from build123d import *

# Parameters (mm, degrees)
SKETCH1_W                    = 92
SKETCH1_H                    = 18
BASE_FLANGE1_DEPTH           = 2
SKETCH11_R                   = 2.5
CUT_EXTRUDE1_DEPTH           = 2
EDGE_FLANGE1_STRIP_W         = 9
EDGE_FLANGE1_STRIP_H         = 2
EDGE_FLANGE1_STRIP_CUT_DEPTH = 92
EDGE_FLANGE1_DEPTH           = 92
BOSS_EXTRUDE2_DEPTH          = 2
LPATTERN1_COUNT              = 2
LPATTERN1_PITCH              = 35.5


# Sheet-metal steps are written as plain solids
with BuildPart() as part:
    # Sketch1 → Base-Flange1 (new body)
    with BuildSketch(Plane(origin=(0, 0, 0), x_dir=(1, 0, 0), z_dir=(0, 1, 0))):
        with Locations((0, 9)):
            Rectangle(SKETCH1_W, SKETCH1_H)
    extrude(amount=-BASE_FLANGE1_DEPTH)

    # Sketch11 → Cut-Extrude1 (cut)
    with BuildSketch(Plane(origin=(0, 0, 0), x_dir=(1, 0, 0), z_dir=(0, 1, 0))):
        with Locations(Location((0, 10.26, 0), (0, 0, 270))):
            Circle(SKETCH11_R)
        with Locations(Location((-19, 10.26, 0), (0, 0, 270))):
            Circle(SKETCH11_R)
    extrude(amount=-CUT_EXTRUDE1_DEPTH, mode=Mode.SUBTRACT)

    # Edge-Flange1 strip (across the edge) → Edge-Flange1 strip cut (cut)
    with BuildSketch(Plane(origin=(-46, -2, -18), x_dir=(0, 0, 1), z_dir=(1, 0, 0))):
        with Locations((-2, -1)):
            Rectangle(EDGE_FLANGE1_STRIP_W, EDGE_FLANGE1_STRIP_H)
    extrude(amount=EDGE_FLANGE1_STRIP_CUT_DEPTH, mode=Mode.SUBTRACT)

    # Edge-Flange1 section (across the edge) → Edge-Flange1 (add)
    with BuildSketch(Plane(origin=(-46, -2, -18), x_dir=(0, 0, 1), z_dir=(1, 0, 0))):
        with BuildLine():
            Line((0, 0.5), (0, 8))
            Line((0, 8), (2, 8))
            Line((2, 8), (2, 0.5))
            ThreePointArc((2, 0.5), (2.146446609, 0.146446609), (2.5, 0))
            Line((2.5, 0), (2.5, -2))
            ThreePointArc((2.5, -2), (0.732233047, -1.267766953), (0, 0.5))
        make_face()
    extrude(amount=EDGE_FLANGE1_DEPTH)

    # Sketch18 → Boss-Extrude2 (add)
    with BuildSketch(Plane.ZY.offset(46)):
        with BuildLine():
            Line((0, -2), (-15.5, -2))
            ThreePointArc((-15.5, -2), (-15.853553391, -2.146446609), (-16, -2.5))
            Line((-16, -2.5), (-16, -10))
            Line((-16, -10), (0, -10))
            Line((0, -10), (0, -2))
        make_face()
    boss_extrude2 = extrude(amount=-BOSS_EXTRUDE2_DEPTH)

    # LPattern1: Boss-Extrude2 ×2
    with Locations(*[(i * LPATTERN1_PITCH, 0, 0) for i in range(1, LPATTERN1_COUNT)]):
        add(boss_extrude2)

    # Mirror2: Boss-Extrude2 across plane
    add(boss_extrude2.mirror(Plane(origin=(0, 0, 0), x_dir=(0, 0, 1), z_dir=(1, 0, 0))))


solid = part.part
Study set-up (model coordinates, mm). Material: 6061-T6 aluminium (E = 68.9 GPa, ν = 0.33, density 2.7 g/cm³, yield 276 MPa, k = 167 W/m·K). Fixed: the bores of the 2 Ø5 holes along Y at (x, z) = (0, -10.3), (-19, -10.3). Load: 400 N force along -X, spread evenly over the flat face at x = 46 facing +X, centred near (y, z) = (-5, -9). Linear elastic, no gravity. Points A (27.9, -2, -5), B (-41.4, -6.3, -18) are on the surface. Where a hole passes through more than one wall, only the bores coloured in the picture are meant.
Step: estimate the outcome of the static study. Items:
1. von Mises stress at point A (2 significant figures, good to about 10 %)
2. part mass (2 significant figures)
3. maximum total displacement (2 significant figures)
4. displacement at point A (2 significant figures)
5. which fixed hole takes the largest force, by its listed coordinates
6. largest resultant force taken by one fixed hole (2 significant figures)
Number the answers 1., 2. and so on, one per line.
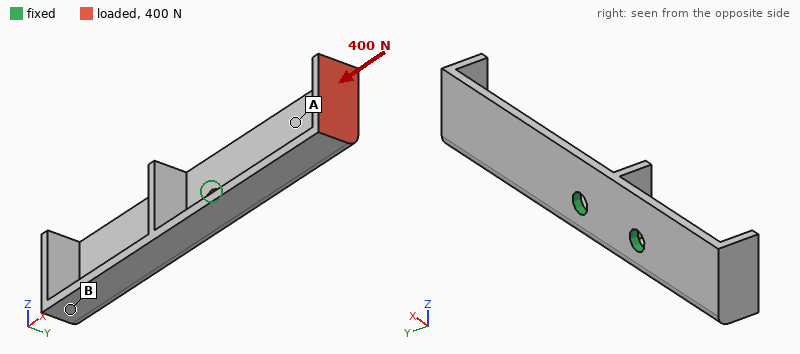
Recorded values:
1. 21 MPa
2. 14 g
3. 0.19 mm
4. 0.046 mm
5. (0, -10.3)
6. 250 N
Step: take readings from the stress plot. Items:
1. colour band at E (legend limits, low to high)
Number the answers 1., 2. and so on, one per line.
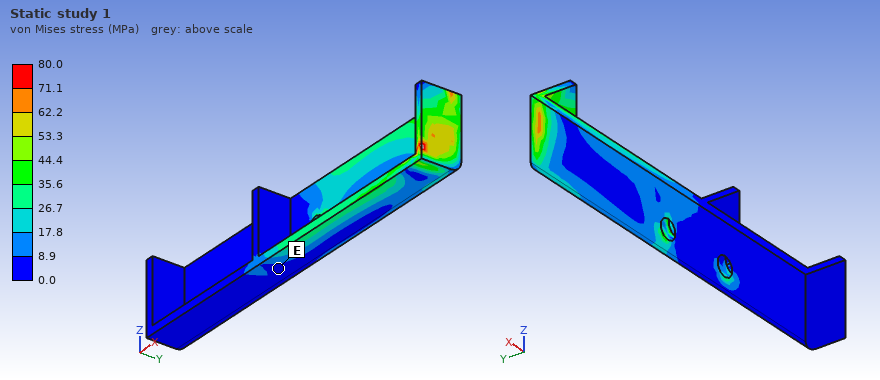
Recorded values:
1. 0.0 to 8.9 MPa
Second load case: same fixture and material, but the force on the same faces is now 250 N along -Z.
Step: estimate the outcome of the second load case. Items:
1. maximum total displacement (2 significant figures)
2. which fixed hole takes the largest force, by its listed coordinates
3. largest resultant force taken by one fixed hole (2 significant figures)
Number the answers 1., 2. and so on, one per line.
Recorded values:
1. 0.44 mm
2. (0, -10.3)
3. 600 N
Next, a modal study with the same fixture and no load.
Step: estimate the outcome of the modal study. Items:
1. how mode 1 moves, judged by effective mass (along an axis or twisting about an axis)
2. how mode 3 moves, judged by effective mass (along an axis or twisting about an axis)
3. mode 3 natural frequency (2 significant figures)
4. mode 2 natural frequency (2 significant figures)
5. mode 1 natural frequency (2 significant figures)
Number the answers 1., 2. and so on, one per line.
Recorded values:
1. along Y
2. along Y
3. 3500 Hz
4. 2700 Hz
5. 1700 Hz
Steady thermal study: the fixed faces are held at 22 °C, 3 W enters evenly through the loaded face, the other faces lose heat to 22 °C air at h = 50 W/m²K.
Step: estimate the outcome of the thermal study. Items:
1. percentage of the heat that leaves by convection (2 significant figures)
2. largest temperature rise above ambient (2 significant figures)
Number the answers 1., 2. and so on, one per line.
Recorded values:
1. 31 %
2. 15 K
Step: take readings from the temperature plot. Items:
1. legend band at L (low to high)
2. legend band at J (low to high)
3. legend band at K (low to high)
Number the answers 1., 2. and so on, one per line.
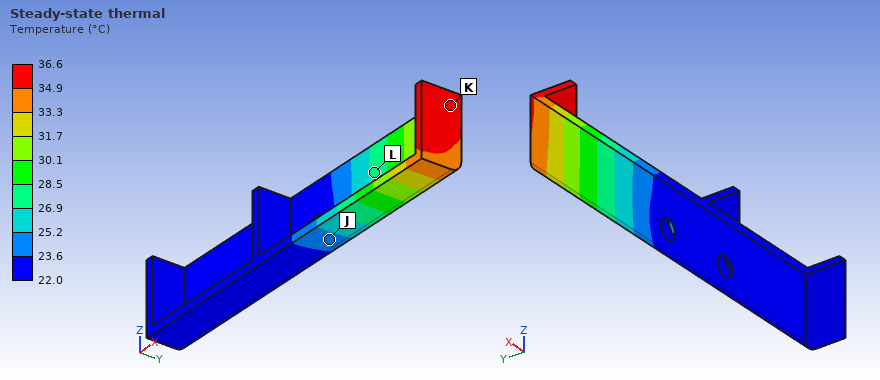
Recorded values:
1. 26.9 to 28.5 °C
2. 23.6 to 25.2 °C
3. 34.9 to 36.6 °C
